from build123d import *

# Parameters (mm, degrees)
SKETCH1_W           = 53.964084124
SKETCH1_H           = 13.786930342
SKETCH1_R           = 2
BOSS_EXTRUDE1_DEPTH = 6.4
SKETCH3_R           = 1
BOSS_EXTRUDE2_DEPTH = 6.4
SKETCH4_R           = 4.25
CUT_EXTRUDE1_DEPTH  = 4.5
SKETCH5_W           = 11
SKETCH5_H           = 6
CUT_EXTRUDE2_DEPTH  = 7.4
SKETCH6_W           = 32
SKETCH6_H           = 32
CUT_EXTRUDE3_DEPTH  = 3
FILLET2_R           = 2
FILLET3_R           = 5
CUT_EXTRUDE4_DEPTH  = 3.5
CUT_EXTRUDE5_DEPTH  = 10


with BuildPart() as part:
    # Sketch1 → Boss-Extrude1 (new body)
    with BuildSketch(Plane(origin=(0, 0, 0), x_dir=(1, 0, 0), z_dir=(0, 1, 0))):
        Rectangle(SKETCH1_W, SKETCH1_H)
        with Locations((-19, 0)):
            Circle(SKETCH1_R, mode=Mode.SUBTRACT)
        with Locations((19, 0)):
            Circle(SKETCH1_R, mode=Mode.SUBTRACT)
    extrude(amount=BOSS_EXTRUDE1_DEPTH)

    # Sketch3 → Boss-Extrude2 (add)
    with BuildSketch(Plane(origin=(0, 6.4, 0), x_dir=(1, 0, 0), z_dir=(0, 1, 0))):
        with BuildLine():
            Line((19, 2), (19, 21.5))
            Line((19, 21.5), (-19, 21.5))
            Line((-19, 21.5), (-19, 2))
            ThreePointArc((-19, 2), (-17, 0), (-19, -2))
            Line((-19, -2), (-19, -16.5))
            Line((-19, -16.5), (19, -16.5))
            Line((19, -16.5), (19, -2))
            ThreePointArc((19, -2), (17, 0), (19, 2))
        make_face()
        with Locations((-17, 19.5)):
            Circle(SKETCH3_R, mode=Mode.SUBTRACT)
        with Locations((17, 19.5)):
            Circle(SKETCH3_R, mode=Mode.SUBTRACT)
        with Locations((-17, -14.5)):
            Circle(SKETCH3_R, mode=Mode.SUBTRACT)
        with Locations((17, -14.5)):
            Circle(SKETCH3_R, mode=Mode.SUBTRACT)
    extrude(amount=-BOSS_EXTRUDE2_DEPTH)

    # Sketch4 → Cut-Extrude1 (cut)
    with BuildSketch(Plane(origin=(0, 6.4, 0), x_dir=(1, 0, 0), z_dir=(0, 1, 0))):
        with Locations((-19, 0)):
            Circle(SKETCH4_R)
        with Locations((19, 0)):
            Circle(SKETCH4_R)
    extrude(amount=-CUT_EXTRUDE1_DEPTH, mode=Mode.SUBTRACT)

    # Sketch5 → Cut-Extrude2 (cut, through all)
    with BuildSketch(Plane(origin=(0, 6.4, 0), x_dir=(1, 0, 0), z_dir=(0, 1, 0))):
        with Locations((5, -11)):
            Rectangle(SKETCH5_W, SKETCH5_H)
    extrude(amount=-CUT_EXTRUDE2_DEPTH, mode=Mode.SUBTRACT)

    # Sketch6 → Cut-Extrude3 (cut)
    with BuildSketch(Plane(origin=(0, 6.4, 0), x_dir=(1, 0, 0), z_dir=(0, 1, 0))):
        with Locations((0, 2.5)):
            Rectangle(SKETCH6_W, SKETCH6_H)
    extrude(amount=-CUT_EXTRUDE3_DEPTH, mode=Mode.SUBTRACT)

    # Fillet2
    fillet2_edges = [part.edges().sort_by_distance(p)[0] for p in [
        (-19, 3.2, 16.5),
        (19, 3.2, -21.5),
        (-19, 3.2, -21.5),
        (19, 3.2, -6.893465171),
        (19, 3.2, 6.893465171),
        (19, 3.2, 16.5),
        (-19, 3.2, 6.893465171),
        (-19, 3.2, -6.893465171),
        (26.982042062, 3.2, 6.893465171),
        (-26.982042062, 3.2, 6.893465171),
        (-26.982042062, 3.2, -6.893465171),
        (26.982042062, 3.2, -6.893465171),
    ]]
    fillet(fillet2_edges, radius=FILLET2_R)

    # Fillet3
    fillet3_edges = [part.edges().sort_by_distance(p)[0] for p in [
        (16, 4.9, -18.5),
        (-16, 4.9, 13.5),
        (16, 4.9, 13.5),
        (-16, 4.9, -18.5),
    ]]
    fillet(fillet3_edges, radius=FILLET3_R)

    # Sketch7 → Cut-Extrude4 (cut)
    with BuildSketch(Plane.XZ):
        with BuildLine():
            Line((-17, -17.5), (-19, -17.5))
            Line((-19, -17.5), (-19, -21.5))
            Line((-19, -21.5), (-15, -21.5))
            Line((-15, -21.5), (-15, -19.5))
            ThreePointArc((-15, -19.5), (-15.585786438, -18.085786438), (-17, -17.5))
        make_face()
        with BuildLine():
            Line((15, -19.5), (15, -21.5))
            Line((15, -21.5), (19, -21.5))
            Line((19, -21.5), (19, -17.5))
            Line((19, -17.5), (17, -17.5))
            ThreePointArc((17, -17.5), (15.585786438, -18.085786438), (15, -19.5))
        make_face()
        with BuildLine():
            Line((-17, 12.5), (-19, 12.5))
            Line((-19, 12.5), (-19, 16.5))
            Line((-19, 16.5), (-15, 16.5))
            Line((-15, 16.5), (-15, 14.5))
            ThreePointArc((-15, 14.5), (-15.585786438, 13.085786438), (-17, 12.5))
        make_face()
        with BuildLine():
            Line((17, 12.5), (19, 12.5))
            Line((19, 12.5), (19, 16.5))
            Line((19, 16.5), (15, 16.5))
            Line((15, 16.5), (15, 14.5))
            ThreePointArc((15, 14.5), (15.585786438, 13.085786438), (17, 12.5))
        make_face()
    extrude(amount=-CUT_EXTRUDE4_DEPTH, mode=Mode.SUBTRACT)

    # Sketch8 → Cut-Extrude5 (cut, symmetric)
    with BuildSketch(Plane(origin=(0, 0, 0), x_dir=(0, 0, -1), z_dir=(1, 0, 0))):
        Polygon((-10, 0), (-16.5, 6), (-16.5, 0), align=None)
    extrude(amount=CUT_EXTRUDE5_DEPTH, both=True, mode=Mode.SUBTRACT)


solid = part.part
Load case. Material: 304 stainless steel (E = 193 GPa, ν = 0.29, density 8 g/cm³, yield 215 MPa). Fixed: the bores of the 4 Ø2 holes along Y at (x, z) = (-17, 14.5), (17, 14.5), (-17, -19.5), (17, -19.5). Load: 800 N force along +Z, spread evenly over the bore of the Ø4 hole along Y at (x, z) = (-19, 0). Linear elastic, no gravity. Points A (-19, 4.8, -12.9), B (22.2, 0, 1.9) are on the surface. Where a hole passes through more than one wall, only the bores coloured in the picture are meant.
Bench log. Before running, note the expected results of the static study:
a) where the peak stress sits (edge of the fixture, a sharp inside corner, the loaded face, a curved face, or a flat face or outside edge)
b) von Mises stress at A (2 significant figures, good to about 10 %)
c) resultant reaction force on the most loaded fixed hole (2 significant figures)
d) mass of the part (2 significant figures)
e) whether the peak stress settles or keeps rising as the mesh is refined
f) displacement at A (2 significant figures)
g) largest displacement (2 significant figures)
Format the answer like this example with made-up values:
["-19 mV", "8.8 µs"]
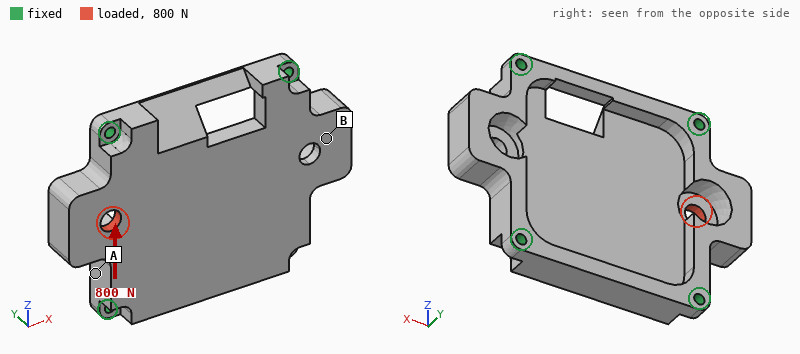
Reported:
["edge of the fixture", "22 MPa", "390 N", "50 g", "keeps rising", "0.77 µm", "3.0 µm"]
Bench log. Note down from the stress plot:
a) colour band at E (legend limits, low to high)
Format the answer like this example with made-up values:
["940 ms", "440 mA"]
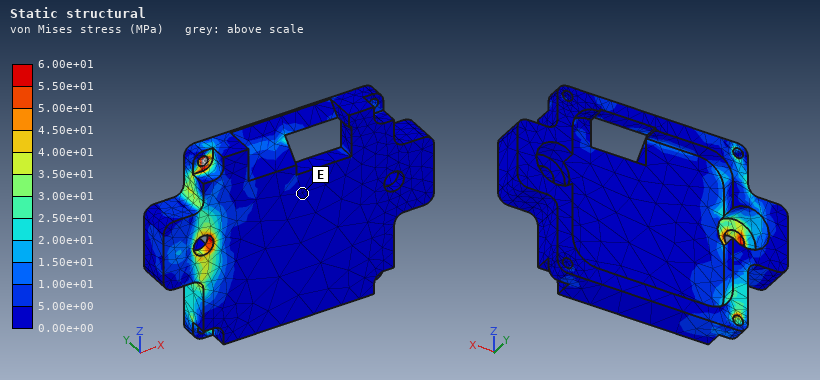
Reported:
["0.00e+00 to 5.00e+00 MPa"]
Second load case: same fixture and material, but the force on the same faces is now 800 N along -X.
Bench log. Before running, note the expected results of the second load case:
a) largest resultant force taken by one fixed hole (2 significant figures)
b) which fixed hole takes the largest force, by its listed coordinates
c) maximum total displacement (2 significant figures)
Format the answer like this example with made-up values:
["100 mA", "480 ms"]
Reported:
["270 N", "(17, -19.5)", "5.5 µm"]
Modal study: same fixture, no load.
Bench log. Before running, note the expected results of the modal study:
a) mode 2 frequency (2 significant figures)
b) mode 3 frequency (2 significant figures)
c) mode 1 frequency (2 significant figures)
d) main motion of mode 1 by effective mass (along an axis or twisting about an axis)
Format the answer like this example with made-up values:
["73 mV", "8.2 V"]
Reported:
["11 kHz", "11 kHz", "10 kHz", "along Y"]
